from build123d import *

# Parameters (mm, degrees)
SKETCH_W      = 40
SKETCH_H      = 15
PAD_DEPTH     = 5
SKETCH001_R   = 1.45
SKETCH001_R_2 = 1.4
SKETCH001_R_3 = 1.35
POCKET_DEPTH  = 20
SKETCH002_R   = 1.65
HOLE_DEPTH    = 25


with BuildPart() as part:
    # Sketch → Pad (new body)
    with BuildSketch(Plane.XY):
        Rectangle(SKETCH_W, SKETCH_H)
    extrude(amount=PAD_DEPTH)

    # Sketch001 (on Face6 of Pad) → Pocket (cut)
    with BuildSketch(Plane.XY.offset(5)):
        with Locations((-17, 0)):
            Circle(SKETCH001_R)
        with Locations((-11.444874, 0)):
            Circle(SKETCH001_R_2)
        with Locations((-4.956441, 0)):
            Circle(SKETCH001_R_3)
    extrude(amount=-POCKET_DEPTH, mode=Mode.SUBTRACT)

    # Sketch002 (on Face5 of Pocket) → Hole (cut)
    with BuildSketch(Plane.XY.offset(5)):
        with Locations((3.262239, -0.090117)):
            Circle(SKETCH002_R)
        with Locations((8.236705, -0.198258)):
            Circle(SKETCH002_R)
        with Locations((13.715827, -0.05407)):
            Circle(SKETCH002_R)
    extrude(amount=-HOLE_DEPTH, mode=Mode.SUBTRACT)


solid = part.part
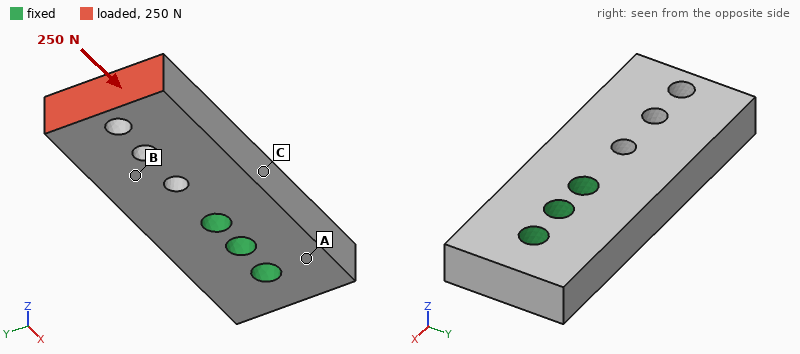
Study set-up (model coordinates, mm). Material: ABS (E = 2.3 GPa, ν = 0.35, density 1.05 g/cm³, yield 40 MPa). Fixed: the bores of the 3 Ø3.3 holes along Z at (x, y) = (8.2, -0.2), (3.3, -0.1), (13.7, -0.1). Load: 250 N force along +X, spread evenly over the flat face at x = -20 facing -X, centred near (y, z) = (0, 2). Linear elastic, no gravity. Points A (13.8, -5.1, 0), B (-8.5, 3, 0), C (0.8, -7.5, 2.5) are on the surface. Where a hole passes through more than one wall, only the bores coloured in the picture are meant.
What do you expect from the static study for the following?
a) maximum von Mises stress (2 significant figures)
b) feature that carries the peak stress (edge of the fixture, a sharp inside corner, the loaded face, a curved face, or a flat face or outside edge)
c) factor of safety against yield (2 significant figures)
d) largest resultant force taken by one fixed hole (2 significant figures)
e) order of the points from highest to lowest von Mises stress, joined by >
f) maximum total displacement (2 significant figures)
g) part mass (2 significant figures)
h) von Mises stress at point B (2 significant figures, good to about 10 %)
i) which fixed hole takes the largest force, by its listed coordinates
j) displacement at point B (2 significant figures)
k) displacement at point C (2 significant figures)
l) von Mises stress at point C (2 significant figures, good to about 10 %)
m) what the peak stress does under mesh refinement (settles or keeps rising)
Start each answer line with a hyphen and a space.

- 12 MPa
- a curved face
- 3.4
- 180 N
- B > C > A
- 49 µm
- 2.9 g
- 4.6 MPa
- (3.3, -0.1)
- 22 µm
- 11 µm
- 2.3 MPa
- settles
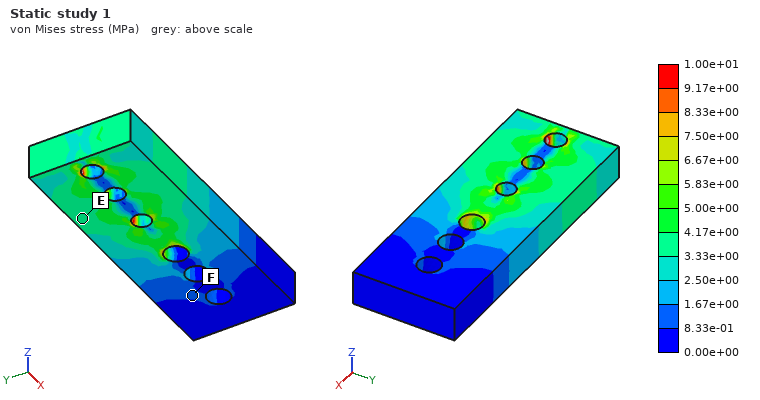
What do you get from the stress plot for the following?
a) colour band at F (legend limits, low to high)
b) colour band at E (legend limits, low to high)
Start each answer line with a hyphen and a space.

- 8.33e-01 to 1.67e+00 MPa
- 3.33e+00 to 4.17e+00 MPa
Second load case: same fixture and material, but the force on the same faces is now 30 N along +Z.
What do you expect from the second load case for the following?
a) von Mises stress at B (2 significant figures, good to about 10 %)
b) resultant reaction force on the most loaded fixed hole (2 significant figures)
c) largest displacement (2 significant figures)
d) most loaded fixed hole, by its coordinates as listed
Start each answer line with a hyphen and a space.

- 6.1 MPa
- 61 N
- 0.39 mm
- (3.3, -0.1)
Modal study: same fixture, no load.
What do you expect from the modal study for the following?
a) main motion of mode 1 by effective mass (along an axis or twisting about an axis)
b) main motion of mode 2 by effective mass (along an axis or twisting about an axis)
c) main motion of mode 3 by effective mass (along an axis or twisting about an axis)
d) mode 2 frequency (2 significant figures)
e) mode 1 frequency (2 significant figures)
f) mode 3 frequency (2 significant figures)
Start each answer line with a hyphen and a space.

- along Z
- along Y
- twisting about X
- 4000 Hz
- 2200 Hz
- 5300 Hz
